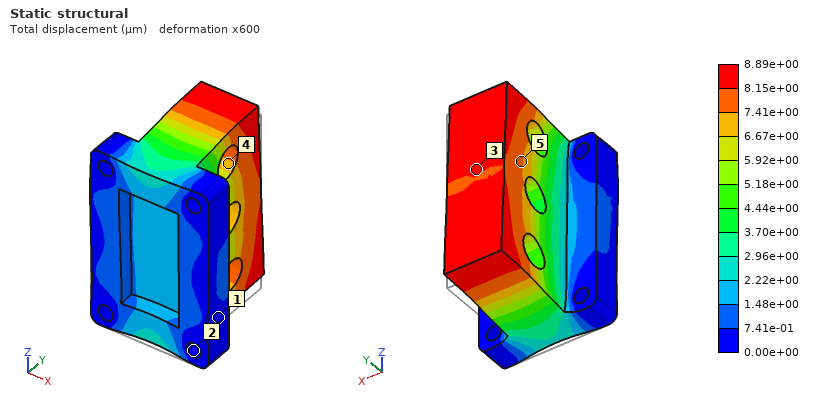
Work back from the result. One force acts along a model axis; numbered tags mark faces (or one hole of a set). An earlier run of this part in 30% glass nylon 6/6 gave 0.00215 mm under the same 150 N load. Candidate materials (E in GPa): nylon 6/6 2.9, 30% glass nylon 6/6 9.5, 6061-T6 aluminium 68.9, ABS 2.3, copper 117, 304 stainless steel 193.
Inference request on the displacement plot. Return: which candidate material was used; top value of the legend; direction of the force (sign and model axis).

ABS
8.89e+00 µm
+Z
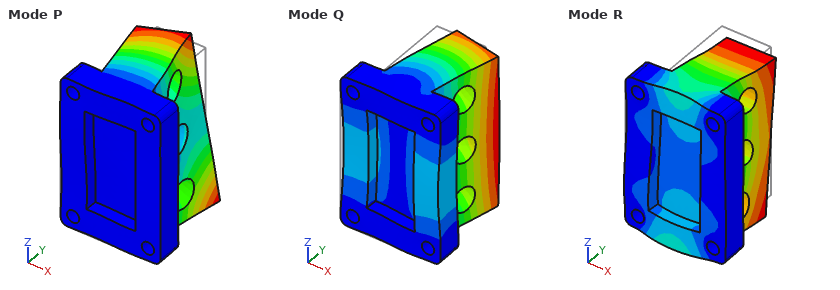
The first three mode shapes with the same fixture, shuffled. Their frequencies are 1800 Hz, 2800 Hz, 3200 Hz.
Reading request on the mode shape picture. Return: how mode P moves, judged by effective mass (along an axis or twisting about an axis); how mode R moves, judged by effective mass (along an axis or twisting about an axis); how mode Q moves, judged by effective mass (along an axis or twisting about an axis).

twisting about Y
along Z
along X
